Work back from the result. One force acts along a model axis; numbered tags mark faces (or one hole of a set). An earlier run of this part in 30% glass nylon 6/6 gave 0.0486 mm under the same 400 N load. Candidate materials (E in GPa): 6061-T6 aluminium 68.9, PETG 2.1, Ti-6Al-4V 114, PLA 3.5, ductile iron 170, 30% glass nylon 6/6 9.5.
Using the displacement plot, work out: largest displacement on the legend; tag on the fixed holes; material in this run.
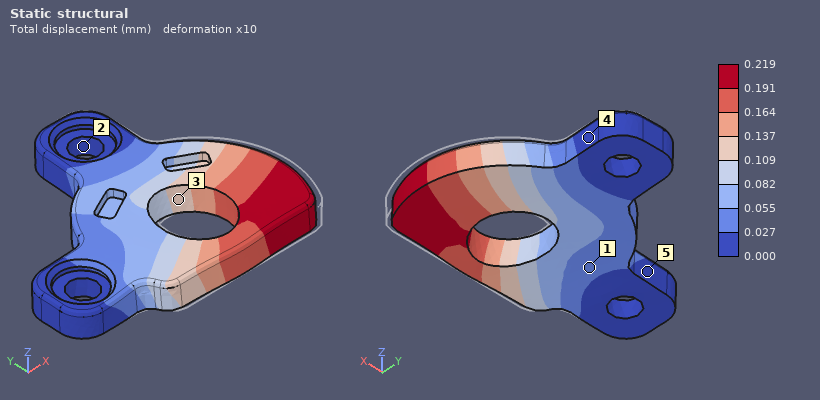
0.219 mm
2
PETG
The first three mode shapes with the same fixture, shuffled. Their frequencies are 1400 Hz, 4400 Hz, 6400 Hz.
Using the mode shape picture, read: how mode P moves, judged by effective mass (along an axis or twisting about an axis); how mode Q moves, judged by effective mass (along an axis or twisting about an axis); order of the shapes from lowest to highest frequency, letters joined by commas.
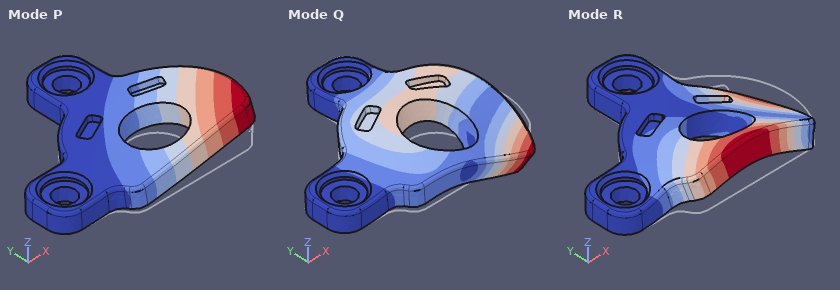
along Z
along Z
P, R, Q
